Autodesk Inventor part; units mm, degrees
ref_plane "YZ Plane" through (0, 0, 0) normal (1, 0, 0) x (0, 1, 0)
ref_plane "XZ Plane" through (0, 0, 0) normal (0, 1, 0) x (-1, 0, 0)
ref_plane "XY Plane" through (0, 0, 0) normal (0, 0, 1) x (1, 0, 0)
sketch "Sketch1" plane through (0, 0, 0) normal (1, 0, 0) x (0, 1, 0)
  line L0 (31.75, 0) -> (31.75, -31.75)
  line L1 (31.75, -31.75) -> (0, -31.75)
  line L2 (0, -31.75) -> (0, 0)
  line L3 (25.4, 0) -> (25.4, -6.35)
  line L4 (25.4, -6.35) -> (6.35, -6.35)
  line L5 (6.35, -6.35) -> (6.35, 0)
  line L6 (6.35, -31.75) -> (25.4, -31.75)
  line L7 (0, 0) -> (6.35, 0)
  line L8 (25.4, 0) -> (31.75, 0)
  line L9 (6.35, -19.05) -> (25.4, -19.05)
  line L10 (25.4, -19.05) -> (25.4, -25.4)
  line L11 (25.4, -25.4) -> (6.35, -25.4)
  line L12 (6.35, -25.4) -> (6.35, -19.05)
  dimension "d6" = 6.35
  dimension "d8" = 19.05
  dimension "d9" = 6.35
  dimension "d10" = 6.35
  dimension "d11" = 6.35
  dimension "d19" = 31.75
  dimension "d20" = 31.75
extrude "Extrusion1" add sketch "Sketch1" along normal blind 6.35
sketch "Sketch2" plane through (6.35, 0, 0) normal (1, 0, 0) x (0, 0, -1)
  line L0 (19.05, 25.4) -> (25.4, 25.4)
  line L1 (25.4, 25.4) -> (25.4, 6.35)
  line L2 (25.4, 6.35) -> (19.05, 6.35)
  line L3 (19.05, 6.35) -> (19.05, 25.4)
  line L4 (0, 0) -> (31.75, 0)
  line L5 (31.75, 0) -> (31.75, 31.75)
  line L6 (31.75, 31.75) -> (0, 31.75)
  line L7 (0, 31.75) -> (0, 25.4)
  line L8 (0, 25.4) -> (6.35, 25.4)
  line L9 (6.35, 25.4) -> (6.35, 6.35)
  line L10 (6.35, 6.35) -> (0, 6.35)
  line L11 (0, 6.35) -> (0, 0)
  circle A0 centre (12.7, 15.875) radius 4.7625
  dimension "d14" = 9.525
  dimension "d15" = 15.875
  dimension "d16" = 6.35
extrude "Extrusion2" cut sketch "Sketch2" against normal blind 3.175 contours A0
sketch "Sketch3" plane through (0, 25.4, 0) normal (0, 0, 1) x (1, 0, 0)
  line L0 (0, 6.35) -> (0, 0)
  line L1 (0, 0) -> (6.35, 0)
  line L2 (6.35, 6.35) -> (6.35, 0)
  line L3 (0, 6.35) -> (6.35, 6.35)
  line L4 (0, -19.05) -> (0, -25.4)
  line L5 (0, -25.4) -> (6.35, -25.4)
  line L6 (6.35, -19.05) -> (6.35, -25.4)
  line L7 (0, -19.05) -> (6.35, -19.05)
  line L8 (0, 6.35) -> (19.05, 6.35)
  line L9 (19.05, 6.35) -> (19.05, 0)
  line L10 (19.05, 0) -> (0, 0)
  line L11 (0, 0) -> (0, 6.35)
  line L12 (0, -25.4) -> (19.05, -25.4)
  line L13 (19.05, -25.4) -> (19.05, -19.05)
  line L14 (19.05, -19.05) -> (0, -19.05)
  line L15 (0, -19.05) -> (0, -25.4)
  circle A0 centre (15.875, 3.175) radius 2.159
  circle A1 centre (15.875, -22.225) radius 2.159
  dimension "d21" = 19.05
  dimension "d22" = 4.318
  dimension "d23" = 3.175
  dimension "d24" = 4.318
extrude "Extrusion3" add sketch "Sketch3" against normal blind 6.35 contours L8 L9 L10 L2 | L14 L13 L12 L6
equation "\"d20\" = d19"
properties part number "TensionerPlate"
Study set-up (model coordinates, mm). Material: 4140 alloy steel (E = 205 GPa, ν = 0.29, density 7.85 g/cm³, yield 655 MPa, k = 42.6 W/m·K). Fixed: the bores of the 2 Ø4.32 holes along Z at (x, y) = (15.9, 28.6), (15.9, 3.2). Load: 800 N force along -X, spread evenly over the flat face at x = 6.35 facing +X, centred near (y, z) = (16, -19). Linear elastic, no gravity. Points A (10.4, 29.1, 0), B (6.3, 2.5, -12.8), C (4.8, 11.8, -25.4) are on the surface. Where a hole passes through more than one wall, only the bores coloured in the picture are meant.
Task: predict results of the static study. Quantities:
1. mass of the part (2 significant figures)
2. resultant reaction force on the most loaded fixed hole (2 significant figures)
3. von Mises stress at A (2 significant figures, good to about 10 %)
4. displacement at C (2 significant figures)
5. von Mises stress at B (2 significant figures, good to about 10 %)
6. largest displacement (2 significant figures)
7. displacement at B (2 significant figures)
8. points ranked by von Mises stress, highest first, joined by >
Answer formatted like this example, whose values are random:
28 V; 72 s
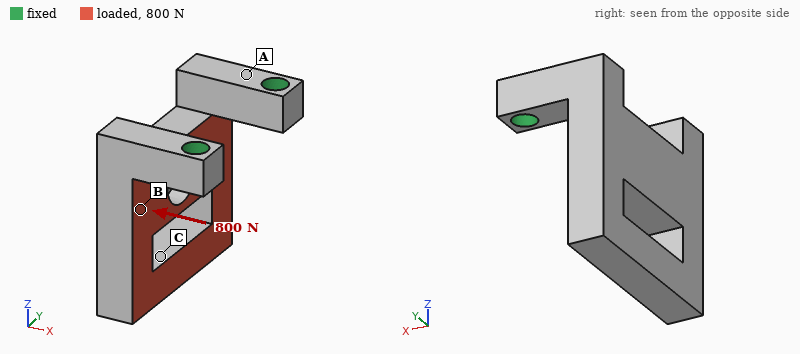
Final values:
43 g; 400 N; 150 MPa; 0.079 mm; 49 MPa; 0.11 mm; 0.029 mm; A > B > C
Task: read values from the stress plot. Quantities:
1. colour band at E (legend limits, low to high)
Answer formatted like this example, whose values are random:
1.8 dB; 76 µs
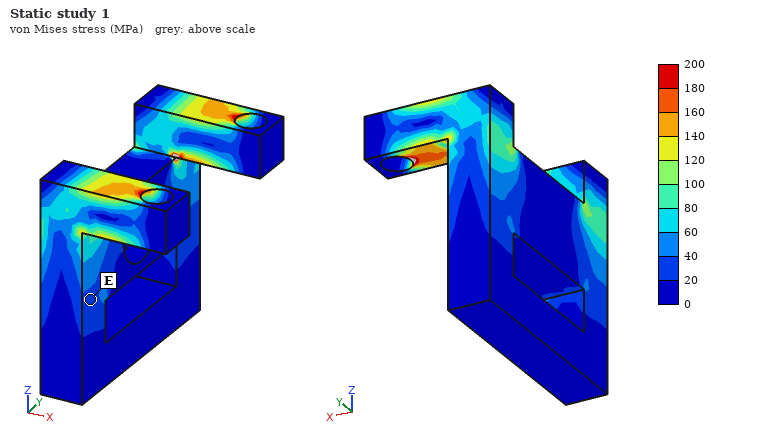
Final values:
20 to 40 MPa
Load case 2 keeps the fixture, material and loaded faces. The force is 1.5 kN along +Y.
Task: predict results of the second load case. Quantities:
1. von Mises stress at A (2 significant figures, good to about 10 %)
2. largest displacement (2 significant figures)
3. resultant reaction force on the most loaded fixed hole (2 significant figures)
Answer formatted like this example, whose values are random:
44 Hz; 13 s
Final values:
90 MPa; 51 µm; 1.1 kN
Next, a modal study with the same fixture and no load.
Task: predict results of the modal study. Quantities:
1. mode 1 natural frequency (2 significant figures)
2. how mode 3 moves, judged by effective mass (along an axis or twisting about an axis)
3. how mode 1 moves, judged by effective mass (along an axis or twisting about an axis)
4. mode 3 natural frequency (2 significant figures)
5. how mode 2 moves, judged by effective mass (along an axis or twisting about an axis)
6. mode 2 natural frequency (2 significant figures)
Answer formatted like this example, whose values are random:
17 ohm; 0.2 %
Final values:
2900 Hz; along Y; along X; 9100 Hz; along Y; 5900 Hz
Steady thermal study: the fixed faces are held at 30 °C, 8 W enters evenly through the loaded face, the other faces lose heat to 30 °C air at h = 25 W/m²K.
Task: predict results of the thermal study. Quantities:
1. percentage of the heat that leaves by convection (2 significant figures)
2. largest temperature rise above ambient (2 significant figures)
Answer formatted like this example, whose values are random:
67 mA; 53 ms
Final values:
22 %; 42 K
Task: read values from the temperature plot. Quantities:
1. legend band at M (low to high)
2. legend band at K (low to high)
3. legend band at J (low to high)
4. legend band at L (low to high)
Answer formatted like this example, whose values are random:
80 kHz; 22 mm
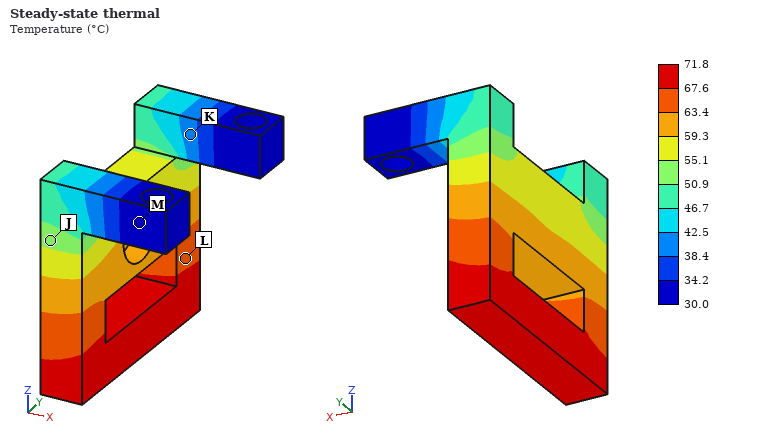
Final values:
30.0 to 34.2 °C; 38.4 to 42.5 °C; 50.9 to 55.1 °C; 63.4 to 67.6 °C
